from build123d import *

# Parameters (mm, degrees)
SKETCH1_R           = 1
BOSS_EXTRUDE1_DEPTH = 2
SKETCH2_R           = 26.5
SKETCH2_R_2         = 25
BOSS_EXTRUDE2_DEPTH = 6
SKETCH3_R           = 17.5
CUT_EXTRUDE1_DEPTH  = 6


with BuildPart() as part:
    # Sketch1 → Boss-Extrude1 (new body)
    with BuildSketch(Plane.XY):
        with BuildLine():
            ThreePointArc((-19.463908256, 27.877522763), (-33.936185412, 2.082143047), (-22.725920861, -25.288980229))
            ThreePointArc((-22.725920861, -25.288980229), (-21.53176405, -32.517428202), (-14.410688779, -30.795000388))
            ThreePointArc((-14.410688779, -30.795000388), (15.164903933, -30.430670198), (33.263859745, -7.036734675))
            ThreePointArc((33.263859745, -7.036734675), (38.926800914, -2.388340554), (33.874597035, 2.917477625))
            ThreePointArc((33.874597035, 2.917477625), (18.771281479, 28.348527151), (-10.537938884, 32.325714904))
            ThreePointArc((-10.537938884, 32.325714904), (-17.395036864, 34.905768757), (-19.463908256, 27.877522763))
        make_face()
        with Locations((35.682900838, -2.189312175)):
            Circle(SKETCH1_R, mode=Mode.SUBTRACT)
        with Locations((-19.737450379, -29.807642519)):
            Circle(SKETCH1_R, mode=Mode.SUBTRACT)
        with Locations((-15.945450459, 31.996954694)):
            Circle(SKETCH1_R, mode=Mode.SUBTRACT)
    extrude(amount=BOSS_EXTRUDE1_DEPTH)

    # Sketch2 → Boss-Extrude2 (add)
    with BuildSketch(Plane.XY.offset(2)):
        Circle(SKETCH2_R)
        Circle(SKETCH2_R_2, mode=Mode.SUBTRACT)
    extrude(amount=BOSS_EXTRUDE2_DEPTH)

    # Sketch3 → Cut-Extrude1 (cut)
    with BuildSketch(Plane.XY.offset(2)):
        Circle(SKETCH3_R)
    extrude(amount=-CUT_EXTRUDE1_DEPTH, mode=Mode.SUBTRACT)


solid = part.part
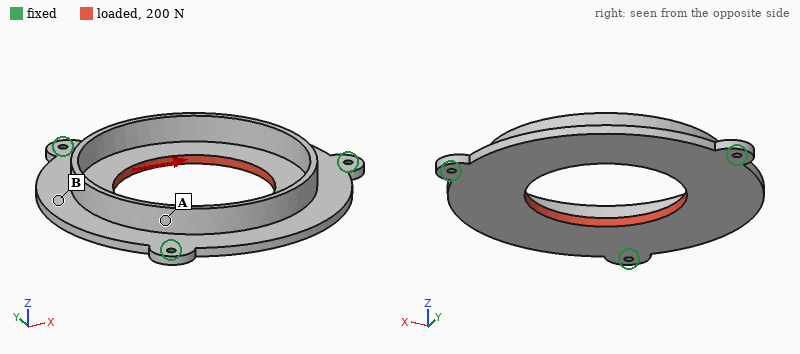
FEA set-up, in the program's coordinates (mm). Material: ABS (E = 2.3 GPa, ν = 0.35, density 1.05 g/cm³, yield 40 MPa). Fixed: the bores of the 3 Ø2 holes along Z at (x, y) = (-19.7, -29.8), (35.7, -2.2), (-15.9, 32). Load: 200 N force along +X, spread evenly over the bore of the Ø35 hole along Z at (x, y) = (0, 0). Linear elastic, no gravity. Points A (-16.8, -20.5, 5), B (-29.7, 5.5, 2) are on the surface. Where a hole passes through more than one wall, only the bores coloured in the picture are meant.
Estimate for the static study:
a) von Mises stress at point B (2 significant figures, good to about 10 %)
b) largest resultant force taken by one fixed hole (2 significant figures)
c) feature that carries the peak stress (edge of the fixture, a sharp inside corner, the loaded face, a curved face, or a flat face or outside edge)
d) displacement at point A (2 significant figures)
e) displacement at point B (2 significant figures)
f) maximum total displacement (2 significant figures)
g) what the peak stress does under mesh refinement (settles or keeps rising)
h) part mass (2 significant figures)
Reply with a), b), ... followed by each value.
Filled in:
a) 2.0 MPa
b) 72 N
c) edge of the fixture
d) 45 µm
e) 76 µm
f) 88 µm
g) keeps rising
h) 7.4 g
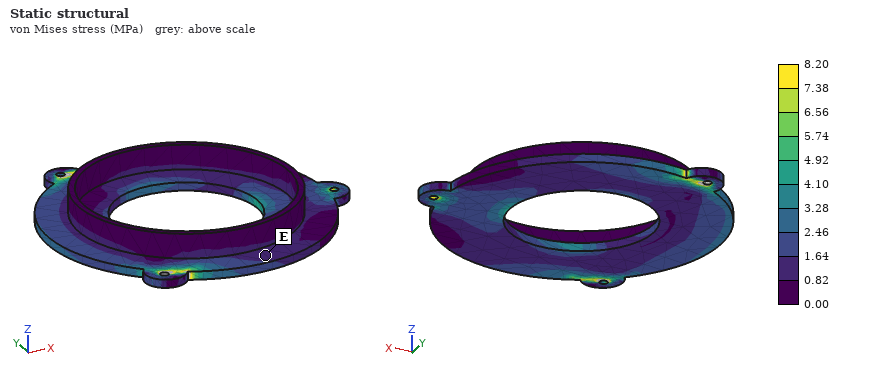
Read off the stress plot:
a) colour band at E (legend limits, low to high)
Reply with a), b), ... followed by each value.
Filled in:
a) 0.82 to 1.64 MPa
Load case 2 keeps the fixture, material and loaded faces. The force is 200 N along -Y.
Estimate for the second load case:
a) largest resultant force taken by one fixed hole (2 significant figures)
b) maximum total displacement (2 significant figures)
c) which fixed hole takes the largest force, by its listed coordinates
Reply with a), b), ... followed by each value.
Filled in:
a) 75 N
b) 80 µm
c) (35.7, -2.2)
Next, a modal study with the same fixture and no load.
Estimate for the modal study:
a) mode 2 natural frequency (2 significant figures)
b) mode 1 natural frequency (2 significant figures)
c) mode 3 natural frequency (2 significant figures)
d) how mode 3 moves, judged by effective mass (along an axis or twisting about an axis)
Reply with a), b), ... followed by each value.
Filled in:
a) 760 Hz
b) 760 Hz
c) 920 Hz
d) along Z
